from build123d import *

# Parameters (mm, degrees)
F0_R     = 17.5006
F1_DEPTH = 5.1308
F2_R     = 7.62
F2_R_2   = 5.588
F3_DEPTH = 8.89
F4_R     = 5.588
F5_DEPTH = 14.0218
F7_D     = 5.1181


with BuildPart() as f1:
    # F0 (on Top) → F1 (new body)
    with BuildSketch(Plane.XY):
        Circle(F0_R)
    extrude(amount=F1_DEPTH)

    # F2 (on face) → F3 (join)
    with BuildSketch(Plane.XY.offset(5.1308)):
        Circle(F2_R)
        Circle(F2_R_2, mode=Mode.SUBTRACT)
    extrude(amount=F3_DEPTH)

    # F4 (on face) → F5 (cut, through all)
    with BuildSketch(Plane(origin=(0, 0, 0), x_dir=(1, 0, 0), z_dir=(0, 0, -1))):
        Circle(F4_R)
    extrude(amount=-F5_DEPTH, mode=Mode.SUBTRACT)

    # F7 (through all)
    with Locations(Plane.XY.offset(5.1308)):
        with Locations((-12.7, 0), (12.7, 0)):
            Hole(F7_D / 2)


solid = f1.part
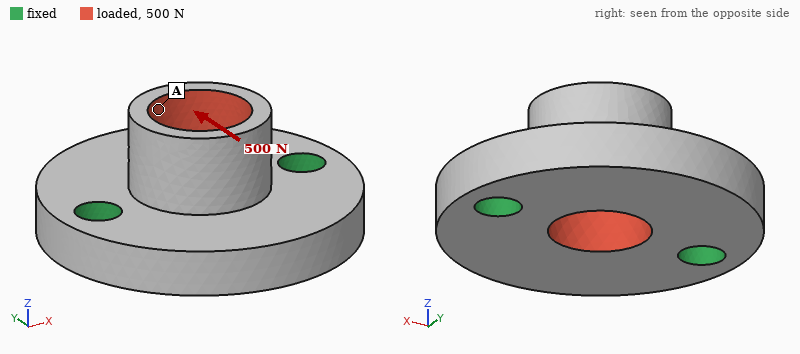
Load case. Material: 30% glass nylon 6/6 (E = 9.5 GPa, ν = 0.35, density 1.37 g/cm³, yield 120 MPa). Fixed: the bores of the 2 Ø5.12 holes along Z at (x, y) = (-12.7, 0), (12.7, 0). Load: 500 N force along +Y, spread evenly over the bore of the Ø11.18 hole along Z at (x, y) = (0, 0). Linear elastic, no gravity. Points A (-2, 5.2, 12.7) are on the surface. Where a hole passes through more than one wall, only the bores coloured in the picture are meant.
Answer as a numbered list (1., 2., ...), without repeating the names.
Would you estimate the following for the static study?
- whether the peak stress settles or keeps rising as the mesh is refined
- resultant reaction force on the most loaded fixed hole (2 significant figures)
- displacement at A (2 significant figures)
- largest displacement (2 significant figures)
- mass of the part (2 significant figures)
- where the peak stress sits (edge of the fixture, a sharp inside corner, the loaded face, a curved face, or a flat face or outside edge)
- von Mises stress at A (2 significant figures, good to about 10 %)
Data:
1. keeps rising
2. 250 N
3. 40 µm
4. 47 µm
5. 6.8 g
6. edge of the fixture
7. 3.6 MPa
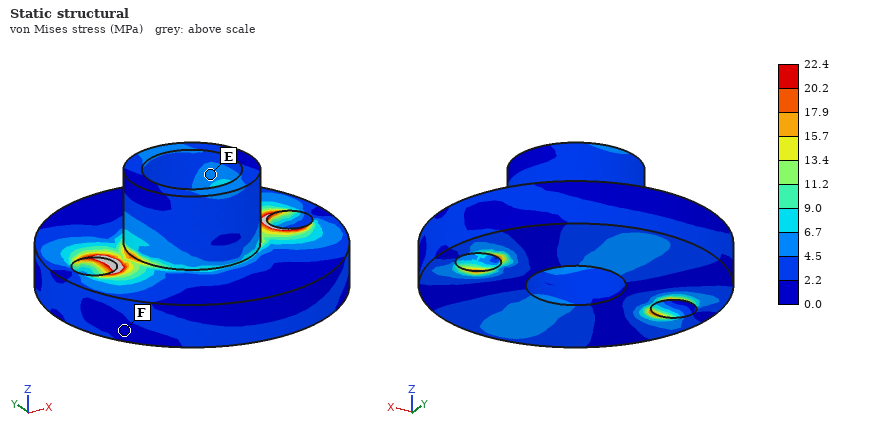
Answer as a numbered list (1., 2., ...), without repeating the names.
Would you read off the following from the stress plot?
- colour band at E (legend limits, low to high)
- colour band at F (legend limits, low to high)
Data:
1. 4.5 to 6.7 MPa
2. 0.0 to 2.2 MPa
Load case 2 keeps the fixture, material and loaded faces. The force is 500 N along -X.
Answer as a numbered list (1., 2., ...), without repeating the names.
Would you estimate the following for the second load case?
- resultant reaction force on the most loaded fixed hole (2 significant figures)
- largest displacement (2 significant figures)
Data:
1. 270 N
2. 21 µm
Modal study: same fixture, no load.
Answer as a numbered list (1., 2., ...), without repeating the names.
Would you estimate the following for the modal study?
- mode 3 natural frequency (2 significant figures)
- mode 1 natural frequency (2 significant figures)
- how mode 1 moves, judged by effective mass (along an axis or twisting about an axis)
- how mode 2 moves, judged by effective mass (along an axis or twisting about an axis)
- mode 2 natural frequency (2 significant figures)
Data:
1. 18 kHz
2. 7100 Hz
3. twisting about X
4. along Z
5. 9100 Hz
